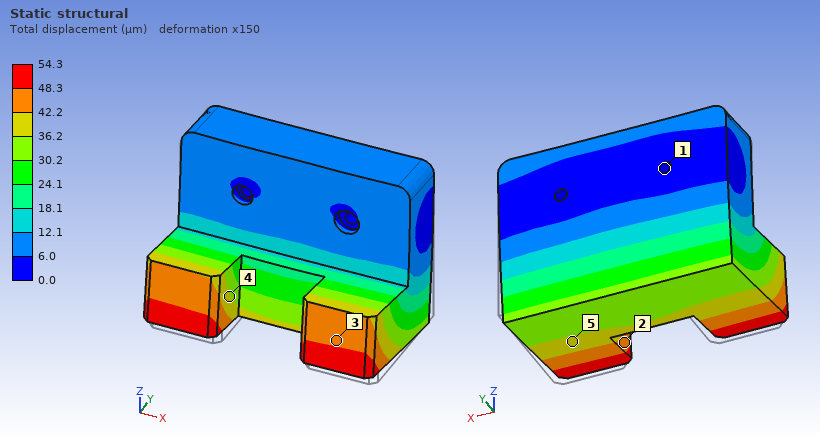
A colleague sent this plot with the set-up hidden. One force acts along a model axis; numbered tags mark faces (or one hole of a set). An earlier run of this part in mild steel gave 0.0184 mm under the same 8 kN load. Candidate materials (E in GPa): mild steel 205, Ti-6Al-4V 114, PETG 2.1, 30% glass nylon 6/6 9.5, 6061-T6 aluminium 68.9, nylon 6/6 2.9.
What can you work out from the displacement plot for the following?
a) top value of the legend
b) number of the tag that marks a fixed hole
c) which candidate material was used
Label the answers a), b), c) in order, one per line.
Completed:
a) 54.3 µm
b) 1
c) 6061-T6 aluminium
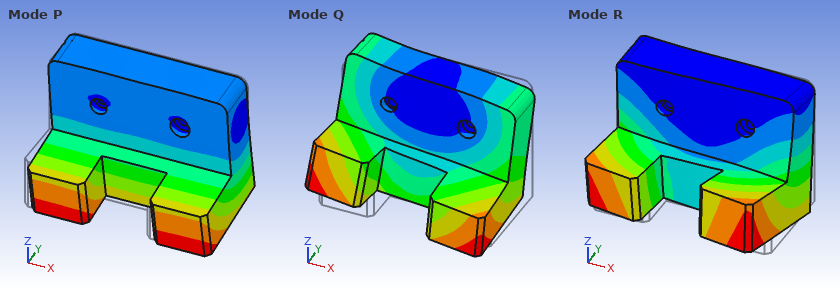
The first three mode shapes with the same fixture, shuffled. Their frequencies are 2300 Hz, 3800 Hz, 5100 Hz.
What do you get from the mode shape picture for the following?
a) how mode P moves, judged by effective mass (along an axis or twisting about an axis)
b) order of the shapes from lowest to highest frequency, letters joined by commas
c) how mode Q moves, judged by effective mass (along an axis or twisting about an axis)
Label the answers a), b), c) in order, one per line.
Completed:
a) along Y
b) P, R, Q
c) along X
